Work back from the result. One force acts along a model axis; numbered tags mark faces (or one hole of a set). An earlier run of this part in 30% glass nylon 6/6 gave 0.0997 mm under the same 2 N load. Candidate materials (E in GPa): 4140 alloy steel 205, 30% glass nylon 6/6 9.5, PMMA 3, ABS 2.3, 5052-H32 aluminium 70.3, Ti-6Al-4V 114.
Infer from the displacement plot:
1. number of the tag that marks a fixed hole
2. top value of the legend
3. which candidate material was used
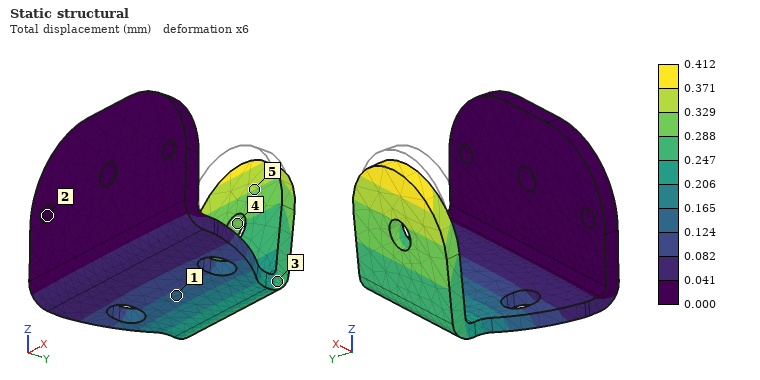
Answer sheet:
2
0.412 mm
ABS
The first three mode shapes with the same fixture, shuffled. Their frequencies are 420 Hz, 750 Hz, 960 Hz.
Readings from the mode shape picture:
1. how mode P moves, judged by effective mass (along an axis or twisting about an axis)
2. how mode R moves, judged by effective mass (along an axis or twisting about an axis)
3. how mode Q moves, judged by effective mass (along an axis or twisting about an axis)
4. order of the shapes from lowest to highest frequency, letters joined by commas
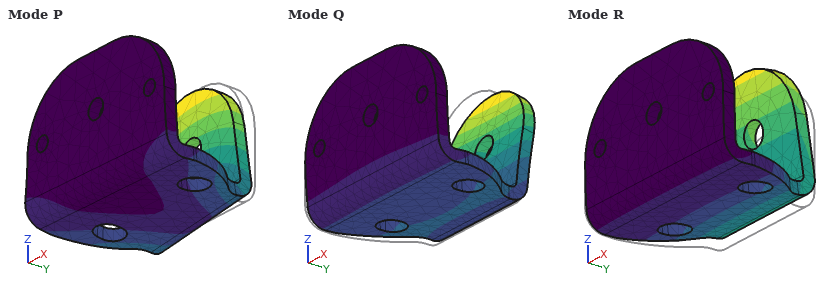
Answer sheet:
along X
along Z
along Y
R, P, Q
